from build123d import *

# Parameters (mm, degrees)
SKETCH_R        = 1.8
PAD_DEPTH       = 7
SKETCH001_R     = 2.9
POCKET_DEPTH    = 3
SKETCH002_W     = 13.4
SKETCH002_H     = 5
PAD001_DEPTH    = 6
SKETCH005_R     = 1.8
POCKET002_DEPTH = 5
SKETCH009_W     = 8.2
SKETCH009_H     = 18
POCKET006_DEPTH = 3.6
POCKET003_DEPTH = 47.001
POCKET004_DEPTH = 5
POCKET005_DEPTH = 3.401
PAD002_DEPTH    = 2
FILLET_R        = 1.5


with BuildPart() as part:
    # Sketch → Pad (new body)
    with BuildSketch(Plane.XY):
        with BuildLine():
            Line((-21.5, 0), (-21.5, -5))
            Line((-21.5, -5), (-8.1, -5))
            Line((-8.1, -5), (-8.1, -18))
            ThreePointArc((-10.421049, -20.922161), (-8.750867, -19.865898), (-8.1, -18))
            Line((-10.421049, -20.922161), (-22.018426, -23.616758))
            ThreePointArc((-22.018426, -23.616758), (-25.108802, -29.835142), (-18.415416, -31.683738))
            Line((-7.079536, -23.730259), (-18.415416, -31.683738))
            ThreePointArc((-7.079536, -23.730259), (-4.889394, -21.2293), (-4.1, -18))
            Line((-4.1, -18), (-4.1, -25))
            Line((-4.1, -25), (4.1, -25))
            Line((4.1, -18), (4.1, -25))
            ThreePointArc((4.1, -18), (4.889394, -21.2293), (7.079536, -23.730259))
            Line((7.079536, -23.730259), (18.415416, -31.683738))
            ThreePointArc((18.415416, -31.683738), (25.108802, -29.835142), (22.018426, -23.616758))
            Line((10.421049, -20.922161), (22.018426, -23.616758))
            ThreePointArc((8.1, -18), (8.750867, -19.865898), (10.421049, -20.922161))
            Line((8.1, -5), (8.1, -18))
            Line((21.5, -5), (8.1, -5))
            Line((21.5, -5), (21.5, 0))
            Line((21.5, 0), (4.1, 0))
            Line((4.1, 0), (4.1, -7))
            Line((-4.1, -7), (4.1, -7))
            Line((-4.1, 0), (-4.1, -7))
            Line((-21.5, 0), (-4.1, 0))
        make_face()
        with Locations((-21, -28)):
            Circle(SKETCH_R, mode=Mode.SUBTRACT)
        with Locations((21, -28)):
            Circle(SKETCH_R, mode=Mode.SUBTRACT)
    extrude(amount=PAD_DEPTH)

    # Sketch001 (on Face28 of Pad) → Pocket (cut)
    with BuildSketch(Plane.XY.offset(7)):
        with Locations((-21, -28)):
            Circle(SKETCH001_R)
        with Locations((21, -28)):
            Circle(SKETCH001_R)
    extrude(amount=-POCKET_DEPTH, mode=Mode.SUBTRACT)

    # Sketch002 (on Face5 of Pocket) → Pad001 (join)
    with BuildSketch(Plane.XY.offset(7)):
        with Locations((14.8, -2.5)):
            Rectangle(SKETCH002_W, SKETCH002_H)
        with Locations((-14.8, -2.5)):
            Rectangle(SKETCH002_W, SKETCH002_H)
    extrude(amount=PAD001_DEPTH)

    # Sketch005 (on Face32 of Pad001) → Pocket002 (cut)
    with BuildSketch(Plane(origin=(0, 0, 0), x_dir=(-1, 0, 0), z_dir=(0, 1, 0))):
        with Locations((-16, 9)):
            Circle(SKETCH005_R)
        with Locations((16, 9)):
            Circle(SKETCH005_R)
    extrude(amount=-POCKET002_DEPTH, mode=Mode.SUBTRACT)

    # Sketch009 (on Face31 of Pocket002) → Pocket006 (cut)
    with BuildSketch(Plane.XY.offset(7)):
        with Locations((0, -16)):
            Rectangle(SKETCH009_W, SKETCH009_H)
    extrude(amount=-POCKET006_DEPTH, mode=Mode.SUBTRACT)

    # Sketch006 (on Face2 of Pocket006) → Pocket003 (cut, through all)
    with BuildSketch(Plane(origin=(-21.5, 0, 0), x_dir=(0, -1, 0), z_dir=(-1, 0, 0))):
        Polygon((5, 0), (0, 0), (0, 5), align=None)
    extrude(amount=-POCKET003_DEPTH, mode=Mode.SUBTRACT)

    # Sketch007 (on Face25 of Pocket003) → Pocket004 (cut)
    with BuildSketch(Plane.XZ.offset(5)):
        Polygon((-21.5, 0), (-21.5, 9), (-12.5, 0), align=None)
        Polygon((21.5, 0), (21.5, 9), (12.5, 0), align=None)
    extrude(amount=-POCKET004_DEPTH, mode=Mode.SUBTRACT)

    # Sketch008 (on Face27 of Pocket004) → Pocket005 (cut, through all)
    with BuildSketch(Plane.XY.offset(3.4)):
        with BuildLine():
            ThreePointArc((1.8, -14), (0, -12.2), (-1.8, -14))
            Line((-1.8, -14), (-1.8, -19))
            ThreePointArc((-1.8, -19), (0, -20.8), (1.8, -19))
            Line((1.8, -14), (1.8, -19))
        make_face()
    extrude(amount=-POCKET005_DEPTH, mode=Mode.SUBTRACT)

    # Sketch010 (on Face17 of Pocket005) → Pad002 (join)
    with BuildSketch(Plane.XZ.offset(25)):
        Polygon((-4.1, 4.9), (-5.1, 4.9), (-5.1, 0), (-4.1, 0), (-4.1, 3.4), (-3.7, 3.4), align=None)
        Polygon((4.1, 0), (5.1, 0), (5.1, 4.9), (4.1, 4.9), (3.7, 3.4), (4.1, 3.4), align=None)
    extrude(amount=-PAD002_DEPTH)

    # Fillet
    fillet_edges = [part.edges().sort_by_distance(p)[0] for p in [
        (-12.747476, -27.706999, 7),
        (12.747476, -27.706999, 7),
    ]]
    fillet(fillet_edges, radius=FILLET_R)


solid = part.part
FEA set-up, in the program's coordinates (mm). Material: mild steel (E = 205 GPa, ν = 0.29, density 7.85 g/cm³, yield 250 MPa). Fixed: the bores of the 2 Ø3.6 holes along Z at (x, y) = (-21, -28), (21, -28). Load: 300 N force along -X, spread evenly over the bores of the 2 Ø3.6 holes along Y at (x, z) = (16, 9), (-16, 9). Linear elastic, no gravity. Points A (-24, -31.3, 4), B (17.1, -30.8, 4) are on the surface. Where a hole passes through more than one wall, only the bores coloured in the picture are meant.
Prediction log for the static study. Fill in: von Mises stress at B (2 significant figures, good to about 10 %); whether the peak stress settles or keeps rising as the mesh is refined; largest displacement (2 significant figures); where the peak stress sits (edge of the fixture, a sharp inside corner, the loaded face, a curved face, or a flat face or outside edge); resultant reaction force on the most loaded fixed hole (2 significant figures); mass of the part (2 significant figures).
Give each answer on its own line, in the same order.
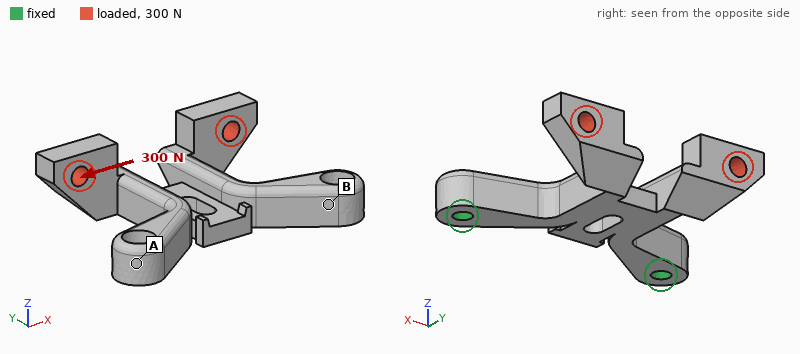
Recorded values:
18 MPa
keeps rising
62 µm
a sharp inside corner
300 N
32 g
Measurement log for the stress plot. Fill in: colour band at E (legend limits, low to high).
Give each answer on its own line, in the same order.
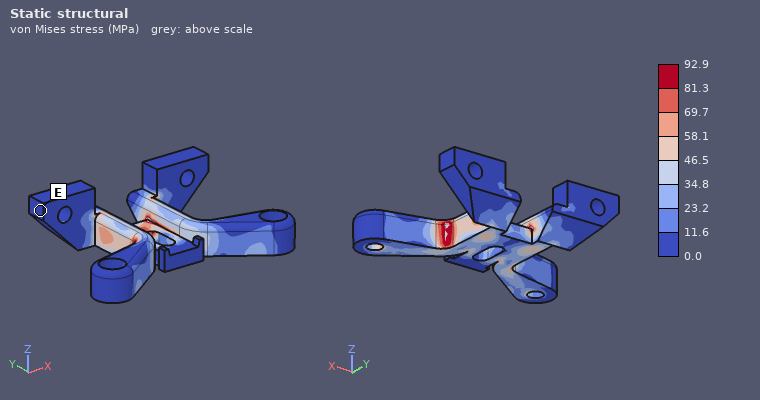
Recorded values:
0.0 to 11.6 MPa
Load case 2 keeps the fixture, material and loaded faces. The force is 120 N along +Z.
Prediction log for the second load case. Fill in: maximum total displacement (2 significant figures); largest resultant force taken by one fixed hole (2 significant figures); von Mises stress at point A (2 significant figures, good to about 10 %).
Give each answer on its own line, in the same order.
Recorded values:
57 µm
62 N
6.6 MPa
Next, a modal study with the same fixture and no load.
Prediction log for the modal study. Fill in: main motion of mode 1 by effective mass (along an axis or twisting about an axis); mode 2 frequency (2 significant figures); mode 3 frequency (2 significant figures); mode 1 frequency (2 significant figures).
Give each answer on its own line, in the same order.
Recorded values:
along Z
3400 Hz
4700 Hz
2500 Hz
